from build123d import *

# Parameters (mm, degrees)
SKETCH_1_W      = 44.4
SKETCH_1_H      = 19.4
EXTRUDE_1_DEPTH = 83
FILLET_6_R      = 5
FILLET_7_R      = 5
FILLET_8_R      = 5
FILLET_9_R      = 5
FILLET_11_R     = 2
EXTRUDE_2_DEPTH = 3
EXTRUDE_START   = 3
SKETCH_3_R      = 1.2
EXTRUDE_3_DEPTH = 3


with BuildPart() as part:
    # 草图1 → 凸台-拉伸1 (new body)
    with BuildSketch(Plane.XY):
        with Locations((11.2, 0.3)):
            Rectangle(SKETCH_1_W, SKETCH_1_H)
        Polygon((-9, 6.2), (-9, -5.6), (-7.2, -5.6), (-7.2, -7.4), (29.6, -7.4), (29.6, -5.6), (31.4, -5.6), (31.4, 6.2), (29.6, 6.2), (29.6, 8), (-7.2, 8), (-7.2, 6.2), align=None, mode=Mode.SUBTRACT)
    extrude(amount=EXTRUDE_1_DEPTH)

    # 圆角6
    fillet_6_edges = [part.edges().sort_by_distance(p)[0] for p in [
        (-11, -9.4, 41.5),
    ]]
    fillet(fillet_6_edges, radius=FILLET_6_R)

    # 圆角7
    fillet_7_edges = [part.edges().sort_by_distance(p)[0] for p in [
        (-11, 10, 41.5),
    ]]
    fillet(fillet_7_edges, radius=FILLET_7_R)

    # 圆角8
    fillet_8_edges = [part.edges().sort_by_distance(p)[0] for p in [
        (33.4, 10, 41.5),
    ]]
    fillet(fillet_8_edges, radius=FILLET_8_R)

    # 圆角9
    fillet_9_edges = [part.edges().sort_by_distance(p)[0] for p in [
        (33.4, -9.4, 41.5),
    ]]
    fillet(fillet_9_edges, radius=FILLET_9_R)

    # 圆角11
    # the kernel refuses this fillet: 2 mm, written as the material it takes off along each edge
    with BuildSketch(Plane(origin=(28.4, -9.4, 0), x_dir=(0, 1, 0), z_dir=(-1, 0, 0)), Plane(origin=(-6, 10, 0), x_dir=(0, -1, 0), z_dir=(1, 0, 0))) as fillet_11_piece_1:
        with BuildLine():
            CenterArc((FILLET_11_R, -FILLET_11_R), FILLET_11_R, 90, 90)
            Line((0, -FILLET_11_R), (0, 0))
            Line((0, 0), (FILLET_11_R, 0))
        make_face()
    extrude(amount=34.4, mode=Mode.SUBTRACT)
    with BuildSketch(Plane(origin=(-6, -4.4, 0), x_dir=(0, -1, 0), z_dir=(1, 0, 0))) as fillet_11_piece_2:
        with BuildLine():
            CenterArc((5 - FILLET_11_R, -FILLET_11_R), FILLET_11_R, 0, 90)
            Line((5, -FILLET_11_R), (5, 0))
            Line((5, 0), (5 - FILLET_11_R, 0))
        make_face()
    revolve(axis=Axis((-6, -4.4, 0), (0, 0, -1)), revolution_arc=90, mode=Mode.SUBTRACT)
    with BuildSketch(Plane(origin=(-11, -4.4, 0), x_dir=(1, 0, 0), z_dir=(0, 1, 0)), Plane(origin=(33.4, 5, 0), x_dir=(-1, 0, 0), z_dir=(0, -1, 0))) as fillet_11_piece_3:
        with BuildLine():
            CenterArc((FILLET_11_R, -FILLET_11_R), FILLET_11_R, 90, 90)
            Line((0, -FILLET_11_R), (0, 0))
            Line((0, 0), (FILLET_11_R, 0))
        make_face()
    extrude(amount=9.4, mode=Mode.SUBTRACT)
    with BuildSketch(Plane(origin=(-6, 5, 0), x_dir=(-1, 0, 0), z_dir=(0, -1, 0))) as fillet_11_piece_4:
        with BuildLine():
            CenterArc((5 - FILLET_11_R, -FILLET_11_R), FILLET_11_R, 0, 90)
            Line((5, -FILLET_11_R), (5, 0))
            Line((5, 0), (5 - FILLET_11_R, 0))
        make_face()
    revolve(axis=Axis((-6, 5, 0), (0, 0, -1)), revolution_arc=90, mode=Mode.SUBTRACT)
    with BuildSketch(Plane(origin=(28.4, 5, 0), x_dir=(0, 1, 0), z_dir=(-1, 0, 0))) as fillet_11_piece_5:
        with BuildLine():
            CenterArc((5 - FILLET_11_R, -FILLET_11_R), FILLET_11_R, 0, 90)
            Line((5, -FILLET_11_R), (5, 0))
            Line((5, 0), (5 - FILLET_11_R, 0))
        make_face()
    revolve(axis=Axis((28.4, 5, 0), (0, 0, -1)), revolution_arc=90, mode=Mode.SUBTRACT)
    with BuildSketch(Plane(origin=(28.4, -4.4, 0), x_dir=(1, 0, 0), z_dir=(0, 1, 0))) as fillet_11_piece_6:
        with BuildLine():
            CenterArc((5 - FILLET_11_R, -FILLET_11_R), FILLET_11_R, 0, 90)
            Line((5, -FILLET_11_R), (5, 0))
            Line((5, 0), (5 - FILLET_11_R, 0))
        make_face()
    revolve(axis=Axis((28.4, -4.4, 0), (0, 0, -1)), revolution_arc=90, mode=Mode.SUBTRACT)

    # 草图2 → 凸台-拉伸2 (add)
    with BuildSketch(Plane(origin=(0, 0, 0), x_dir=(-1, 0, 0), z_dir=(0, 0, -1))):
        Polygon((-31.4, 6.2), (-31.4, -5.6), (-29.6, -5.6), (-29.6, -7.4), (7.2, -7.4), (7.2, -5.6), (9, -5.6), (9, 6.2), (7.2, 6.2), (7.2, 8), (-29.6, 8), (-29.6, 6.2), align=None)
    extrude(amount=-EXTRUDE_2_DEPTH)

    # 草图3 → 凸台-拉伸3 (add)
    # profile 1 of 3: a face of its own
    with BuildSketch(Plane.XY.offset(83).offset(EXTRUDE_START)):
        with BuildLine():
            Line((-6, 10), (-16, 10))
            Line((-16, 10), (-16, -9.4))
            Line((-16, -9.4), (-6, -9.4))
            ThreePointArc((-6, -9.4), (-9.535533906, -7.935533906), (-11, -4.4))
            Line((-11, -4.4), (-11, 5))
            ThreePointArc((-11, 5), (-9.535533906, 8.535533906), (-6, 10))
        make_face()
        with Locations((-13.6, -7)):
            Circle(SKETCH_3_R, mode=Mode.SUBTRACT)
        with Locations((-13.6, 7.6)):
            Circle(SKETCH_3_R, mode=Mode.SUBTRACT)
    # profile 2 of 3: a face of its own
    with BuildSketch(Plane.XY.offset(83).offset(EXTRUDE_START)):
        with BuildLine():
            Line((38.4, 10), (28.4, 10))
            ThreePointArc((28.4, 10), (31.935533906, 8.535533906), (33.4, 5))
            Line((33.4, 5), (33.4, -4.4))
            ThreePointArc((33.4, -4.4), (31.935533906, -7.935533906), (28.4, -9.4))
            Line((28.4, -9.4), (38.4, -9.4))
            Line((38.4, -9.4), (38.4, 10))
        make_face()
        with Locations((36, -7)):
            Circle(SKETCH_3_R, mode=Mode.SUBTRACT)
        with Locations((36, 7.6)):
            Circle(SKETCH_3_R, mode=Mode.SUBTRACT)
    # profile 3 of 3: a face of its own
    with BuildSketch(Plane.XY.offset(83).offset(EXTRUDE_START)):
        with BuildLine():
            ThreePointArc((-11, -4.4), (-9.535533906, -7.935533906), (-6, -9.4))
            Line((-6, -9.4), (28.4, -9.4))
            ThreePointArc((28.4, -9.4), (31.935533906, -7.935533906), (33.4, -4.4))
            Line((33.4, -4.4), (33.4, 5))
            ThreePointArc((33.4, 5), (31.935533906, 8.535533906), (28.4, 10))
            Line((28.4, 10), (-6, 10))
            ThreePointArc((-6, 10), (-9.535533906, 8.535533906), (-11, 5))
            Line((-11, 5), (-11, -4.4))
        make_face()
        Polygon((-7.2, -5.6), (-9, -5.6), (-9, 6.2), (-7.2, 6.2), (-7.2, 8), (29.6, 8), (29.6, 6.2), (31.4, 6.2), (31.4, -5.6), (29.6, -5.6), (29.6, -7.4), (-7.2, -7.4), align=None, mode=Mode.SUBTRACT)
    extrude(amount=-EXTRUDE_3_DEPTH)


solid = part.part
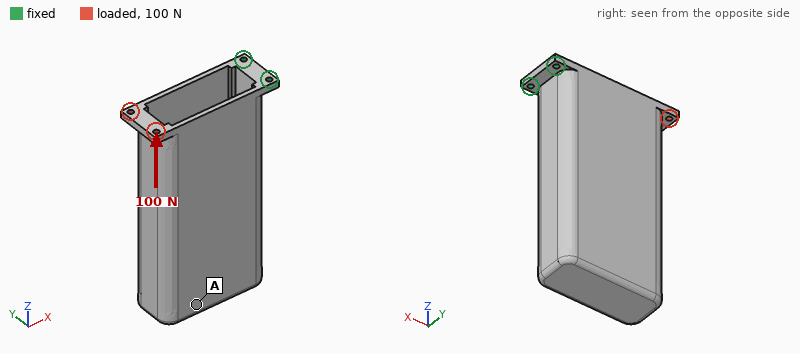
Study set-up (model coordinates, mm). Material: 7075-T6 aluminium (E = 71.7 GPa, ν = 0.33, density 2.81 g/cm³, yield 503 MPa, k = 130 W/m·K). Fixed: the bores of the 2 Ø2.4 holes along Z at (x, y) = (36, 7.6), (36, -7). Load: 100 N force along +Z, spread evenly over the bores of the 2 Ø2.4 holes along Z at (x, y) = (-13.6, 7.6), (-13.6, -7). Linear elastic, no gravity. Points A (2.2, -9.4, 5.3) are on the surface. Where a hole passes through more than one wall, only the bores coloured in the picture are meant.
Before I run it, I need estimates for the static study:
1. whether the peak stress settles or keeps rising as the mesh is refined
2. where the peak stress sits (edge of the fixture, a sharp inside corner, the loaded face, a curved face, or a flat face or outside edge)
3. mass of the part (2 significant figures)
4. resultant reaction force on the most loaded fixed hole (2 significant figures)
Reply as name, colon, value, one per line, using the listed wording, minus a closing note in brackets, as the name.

whether the peak stress settles or keeps rising as the mesh is refined: keeps rising
where the peak stress sits: edge of the fixture
mass of the part: 62 g
resultant reaction force on the most loaded fixed hole: 120 N
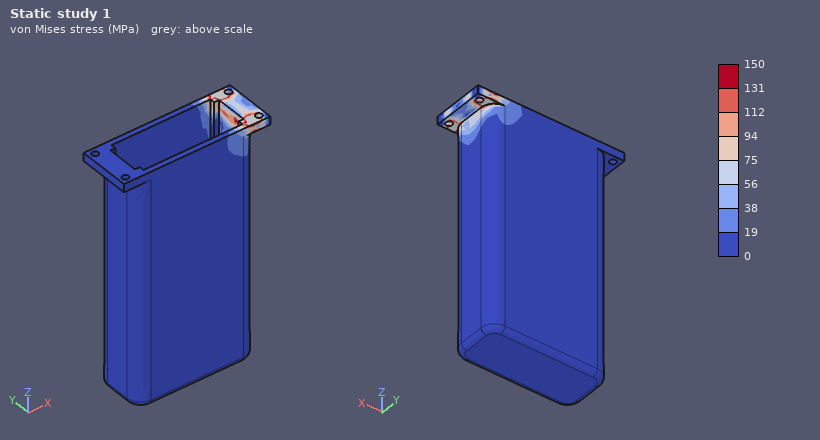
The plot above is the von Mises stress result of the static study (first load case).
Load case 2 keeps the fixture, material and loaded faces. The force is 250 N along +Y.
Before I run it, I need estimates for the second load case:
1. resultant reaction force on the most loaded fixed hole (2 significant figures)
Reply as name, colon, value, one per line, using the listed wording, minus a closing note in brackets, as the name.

resultant reaction force on the most loaded fixed hole: 770 N
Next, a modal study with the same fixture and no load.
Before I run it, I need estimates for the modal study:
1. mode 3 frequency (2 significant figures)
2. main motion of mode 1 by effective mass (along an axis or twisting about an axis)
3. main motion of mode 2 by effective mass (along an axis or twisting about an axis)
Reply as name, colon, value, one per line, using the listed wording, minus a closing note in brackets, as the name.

mode 3 frequency: 1000 Hz
main motion of mode 1 by effective mass: along X
main motion of mode 2 by effective mass: along Y
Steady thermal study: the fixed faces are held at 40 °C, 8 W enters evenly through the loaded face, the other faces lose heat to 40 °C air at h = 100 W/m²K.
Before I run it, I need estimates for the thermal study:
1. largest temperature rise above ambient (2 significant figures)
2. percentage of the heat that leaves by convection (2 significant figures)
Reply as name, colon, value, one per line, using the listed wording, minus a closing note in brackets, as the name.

largest temperature rise above ambient: 25 K
percentage of the heat that leaves by convection: 84 %
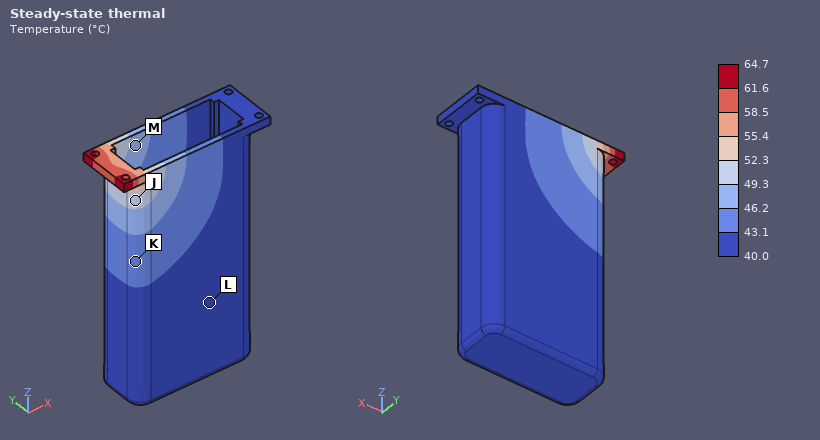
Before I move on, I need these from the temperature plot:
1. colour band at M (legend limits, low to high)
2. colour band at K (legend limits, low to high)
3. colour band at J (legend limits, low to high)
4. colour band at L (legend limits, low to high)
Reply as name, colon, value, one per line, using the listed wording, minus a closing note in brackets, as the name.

colour band at M: 46.2 to 49.3 °C
colour band at K: 43.1 to 46.2 °C
colour band at J: 49.3 to 52.3 °C
colour band at L: 40.0 to 43.1 °C
